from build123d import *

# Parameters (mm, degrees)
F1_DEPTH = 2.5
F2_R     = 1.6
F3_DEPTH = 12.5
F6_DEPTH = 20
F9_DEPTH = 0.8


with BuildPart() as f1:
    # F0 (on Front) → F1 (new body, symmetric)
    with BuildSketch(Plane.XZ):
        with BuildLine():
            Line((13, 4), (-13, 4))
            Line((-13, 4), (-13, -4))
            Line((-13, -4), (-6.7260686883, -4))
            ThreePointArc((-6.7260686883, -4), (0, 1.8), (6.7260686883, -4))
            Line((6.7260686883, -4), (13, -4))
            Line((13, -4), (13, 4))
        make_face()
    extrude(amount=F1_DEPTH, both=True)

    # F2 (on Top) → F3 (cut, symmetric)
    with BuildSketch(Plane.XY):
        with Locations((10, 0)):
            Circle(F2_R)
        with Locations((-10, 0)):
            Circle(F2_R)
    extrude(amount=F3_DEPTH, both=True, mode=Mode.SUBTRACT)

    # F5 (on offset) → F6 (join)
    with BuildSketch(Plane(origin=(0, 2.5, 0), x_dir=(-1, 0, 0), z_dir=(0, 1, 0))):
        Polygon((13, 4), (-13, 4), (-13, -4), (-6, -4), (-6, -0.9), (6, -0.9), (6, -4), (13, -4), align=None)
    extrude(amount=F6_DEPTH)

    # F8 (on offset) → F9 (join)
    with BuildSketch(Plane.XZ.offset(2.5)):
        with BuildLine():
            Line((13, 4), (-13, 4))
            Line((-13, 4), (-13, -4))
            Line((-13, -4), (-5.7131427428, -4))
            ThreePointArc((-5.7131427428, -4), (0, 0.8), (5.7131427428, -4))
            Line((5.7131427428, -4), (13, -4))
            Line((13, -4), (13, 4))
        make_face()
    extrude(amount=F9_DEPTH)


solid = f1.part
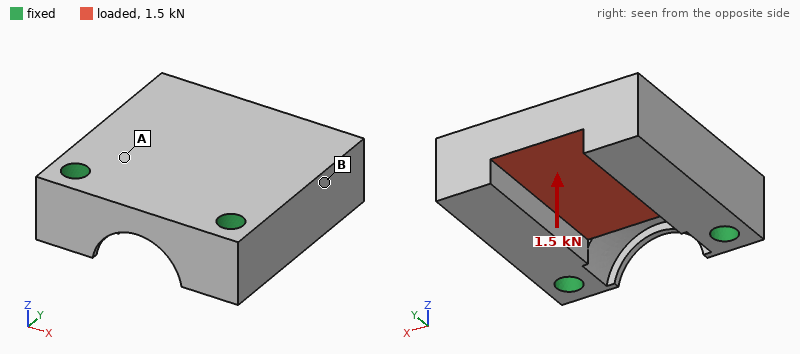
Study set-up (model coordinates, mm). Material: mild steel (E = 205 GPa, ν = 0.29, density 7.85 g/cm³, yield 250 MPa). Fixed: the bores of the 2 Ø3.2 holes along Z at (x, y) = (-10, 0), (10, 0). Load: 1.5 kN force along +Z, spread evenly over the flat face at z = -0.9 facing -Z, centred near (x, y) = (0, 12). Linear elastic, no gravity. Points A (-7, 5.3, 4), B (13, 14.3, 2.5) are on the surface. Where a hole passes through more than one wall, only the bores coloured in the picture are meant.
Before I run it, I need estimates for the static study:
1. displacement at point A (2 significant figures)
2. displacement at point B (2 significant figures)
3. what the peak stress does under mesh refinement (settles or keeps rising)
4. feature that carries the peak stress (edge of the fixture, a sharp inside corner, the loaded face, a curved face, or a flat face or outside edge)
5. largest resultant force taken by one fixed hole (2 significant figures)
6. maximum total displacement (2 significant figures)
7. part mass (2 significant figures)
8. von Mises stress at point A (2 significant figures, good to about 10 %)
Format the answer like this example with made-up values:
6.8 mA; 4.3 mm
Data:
3.6 µm; 8.6 µm; keeps rising; edge of the fixture; 750 N; 21 µm; 33 g; 55 MPa
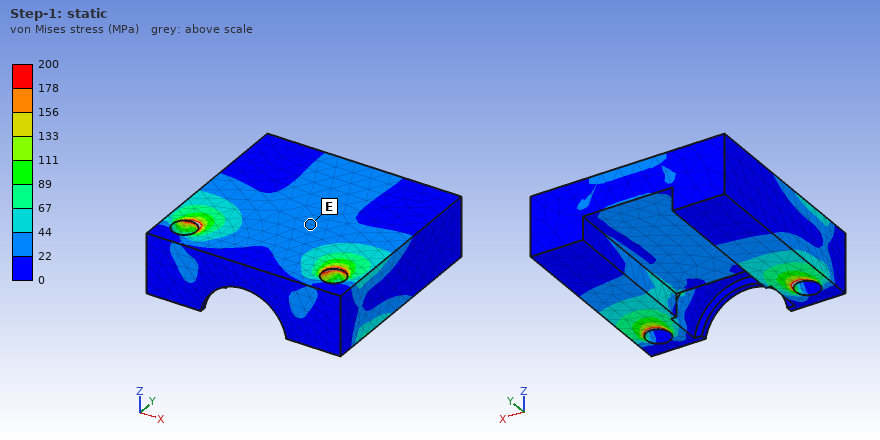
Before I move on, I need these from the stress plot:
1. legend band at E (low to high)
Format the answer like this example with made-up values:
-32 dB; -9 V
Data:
22 to 44 MPa
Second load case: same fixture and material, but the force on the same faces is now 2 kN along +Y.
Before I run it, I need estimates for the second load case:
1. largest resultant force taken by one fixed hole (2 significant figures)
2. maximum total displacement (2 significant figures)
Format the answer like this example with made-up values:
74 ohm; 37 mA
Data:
1.0 kN; 5.0 µm
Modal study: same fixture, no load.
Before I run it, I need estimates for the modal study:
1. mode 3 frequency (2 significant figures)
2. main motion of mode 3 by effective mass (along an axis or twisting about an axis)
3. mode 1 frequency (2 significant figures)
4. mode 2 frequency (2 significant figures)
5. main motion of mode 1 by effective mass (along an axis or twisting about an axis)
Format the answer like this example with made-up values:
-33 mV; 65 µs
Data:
25 kHz; along X; 11 kHz; 18 kHz; along Z
